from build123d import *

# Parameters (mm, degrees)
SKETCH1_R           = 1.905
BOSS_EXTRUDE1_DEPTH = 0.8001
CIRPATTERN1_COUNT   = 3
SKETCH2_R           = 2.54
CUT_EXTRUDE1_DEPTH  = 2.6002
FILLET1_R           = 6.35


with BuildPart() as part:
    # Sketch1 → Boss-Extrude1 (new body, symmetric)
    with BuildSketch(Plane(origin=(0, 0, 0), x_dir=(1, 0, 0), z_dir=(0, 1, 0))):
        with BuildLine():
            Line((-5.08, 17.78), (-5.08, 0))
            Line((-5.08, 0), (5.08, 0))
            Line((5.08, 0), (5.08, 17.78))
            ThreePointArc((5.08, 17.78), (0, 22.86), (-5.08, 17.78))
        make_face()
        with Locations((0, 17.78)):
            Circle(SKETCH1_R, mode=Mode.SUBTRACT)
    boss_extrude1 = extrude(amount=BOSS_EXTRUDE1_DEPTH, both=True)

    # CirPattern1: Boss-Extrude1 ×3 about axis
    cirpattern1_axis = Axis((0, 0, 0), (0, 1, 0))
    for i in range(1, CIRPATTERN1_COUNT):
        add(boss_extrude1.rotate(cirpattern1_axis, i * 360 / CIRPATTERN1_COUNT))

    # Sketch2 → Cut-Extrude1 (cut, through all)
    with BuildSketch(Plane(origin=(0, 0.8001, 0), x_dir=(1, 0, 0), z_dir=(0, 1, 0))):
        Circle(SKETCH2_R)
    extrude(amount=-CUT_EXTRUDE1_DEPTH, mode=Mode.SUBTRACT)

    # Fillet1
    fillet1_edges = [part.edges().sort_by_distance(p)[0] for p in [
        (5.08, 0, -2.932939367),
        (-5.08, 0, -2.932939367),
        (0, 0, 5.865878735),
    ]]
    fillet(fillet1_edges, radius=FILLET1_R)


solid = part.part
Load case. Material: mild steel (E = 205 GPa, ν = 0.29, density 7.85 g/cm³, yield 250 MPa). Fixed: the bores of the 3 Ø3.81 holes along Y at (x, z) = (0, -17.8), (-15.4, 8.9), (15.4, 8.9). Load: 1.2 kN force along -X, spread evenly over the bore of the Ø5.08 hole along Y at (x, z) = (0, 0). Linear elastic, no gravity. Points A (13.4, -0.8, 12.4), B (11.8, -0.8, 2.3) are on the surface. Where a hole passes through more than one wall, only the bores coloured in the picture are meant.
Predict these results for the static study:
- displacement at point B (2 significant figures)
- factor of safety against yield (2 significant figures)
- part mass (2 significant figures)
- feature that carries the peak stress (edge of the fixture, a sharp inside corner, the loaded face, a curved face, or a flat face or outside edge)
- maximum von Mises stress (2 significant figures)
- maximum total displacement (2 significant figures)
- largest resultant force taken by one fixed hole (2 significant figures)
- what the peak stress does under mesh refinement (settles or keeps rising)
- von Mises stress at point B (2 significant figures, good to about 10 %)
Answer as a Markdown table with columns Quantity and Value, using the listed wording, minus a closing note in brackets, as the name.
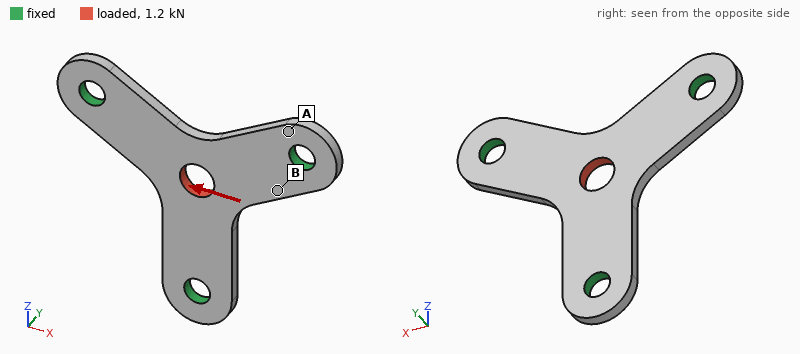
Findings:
| Quantity | Value |
|---|---|
| displacement at point B | 2.1 µm |
| factor of safety against yield | 2.1 |
| part mass | 7.2 g |
| feature that carries the peak stress | the loaded face |
| maximum von Mises stress | 120 MPa |
| maximum total displacement | 5.6 µm |
| largest resultant force taken by one fixed hole | 610 N |
| what the peak stress does under mesh refinement | settles |
| von Mises stress at point B | 42 MPa |
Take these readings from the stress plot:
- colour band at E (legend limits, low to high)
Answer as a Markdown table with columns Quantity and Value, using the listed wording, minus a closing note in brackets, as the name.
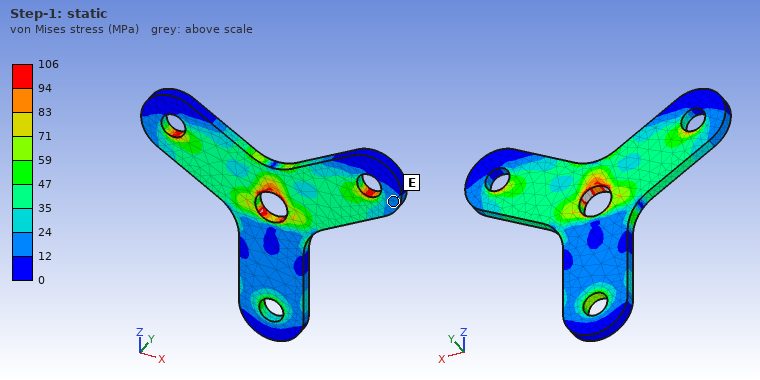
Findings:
| Quantity | Value |
|---|---|
| colour band at E | 12 to 24 MPa |
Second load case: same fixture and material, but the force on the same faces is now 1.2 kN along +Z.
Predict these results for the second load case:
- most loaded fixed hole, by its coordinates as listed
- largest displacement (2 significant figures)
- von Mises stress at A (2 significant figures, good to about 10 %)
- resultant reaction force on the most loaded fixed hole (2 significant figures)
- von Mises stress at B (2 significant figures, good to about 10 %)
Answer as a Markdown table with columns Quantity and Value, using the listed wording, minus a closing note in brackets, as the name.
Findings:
| Quantity | Value |
|---|---|
| most loaded fixed hole, by its coordinates as listed | (0, -17.8) |
| largest displacement | 5.8 µm |
| von Mises stress at A | 25 MPa |
| resultant reaction force on the most loaded fixed hole | 700 N |
| von Mises stress at B | 13 MPa |
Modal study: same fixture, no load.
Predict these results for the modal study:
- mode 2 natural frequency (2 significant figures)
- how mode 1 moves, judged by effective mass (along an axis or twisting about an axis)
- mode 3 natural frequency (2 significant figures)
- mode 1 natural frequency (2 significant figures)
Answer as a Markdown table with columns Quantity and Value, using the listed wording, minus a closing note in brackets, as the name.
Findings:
| Quantity | Value |
|---|---|
| mode 2 natural frequency | 19 kHz |
| how mode 1 moves, judged by effective mass | along Y |
| mode 3 natural frequency | 19 kHz |
| mode 1 natural frequency | 9300 Hz |
